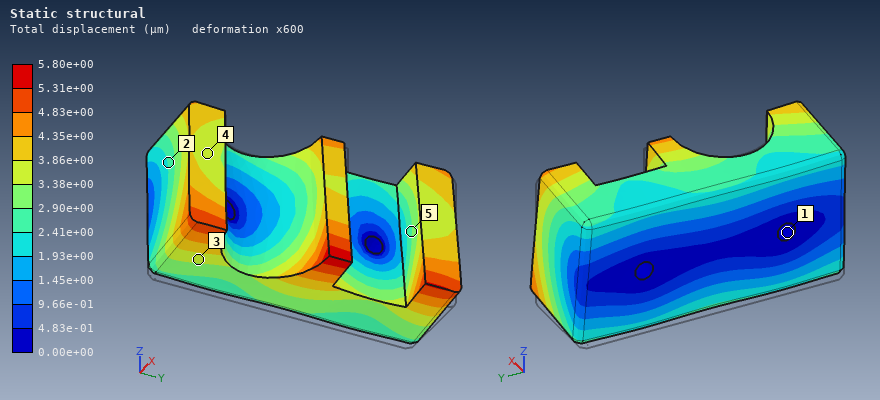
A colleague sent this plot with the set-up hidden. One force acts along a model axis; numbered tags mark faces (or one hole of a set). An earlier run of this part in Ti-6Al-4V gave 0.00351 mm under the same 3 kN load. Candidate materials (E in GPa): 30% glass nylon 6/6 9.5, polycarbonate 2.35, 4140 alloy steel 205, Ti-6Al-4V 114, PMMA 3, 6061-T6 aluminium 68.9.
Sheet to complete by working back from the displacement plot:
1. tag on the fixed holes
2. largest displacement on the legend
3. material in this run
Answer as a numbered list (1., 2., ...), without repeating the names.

1. 1
2. 5.80e+00 µm
3. 6061-T6 aluminium
